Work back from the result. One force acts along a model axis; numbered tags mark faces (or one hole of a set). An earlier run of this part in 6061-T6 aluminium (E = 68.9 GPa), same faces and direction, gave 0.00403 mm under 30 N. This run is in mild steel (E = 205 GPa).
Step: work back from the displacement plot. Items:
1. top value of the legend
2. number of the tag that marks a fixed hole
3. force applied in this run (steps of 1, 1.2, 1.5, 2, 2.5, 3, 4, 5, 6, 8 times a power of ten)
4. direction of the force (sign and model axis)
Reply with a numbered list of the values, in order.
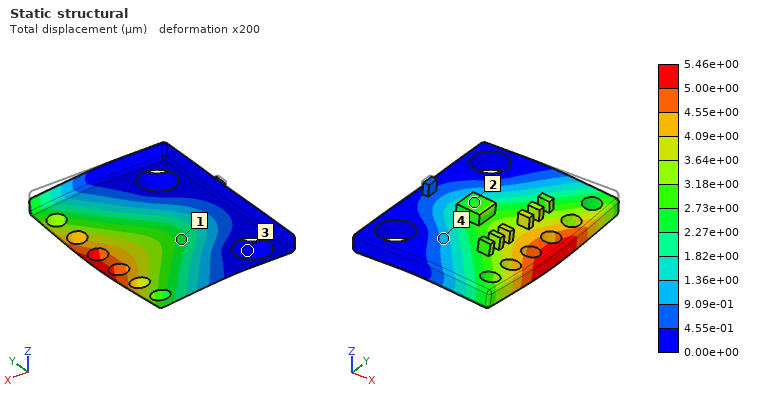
1. 5.46e+00 µm
2. 3
3. 120 N
4. -Z
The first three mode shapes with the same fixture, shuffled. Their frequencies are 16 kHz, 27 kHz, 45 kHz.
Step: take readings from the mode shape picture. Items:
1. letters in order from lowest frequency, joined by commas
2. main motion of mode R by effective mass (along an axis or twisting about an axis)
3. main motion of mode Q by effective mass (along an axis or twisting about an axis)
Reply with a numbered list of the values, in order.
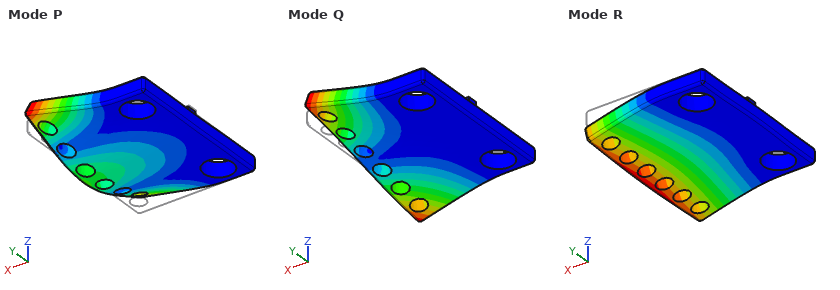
1. R, Q, P
2. along Z
3. twisting about X
